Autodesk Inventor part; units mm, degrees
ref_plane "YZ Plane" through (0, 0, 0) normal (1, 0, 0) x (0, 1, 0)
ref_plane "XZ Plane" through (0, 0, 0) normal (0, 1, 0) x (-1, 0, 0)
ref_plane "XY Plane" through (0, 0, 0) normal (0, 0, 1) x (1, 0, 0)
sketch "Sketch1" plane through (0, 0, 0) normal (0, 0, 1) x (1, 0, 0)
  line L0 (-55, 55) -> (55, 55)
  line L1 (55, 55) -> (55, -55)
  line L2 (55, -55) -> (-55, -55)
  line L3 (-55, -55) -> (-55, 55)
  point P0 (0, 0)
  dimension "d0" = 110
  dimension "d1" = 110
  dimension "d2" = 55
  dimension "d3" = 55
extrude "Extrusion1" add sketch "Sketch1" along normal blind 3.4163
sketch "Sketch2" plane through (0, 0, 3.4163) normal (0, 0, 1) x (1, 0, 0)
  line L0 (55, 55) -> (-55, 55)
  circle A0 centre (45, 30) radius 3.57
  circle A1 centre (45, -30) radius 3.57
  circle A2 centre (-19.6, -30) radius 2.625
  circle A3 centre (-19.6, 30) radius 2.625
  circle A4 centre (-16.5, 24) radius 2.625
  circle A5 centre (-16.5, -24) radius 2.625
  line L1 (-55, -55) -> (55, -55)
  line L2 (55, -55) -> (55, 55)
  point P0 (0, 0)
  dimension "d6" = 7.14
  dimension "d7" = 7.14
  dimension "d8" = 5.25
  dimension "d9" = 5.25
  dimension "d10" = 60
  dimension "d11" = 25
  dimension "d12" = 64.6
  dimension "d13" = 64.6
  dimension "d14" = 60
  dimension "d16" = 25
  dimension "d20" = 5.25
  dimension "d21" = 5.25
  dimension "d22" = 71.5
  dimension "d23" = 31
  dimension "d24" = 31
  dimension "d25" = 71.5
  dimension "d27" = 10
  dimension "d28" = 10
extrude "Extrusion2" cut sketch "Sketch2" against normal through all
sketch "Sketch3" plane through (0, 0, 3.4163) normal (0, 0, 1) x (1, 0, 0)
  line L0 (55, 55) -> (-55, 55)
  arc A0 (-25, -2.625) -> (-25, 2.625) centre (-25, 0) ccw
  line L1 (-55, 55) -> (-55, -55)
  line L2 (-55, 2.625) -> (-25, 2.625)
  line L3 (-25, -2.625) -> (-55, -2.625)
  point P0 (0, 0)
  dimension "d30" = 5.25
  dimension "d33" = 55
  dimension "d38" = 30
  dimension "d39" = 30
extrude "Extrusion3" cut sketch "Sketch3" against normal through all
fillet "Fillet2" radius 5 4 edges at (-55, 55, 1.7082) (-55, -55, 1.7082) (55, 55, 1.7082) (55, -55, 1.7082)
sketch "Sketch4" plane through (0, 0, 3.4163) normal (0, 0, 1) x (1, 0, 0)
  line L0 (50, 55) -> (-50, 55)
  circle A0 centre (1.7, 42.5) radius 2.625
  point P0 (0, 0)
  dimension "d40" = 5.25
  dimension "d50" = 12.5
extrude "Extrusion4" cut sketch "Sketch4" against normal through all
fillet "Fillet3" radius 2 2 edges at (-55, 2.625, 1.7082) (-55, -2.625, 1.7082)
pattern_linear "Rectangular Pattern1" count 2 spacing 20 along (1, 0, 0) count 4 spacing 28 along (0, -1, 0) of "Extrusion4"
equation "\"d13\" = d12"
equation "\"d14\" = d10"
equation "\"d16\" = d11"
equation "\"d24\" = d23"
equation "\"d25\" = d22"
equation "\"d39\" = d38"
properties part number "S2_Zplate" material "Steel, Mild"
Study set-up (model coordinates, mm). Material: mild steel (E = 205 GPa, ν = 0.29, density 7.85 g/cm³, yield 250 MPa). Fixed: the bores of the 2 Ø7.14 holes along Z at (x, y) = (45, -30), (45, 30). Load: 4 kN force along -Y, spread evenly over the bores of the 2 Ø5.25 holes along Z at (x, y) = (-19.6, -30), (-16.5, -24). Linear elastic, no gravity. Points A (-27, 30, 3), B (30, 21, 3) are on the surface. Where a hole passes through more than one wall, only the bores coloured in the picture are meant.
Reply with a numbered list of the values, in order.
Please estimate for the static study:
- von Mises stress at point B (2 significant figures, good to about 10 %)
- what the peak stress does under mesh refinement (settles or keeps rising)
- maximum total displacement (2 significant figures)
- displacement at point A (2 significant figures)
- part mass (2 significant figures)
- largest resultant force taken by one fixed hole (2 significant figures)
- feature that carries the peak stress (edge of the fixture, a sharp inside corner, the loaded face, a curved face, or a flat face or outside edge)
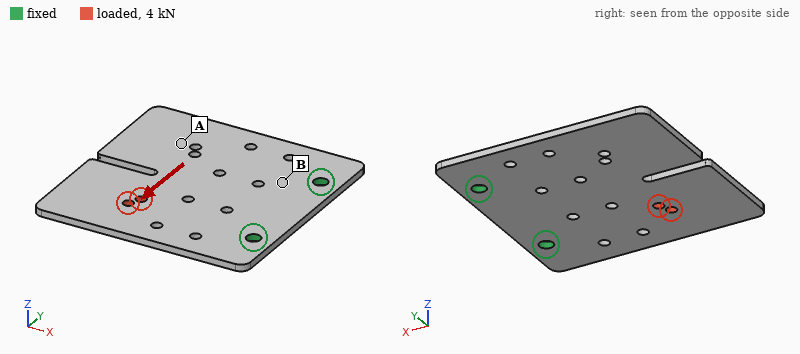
1. 41 MPa
2. keeps rising
3. 40 µm
4. 24 µm
5. 310 g
6. 4.4 kN
7. edge of the fixture
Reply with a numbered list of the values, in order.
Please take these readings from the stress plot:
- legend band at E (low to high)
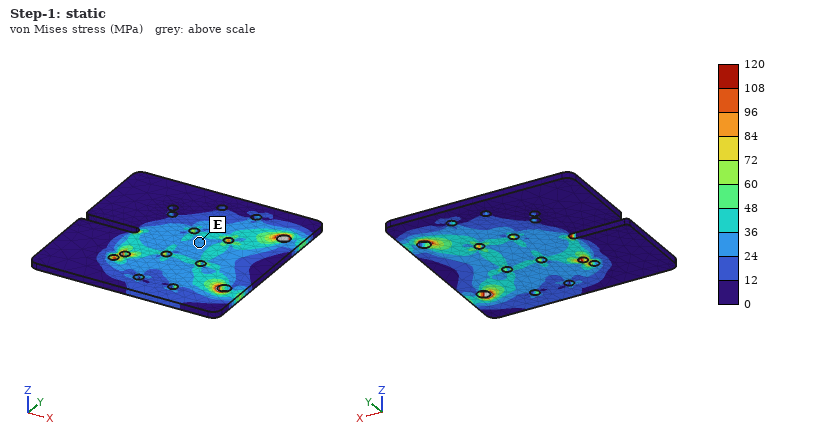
1. 24 to 36 MPa
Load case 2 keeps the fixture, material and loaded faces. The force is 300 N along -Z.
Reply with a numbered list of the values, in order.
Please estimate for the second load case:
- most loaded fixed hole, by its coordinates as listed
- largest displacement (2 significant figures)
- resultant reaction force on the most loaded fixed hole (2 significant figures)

1. (45, -30)
2. 0.88 mm
3. 260 N
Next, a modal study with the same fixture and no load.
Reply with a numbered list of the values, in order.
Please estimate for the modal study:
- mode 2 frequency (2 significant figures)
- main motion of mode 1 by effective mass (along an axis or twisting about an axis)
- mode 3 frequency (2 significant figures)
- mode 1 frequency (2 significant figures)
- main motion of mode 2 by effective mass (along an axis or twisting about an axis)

1. 550 Hz
2. along Z
3. 1400 Hz
4. 280 Hz
5. twisting about X
